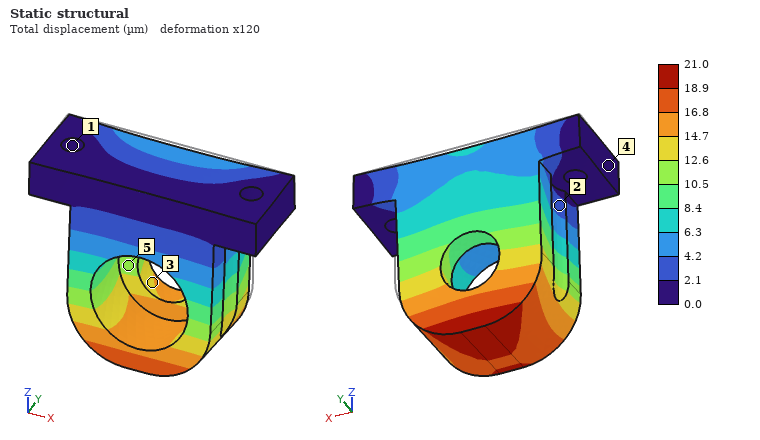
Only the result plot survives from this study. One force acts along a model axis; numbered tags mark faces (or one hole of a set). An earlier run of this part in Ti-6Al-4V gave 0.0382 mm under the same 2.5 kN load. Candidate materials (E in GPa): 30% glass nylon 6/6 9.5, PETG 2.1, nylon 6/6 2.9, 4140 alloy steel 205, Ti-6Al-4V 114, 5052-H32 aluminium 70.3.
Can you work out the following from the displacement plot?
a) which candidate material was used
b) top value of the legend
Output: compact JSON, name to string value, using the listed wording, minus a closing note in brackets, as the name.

{"which candidate material was used": "4140 alloy steel", "top value of the legend": "21.0 µm"}
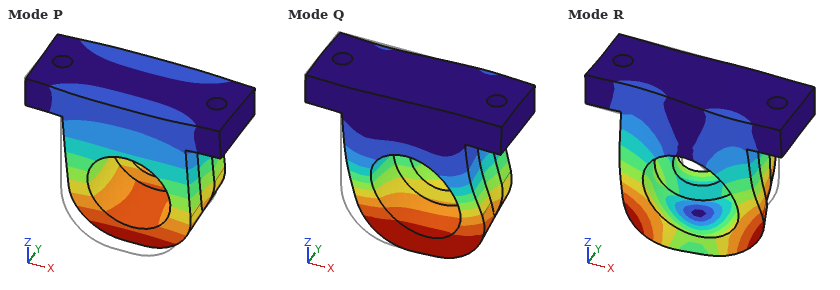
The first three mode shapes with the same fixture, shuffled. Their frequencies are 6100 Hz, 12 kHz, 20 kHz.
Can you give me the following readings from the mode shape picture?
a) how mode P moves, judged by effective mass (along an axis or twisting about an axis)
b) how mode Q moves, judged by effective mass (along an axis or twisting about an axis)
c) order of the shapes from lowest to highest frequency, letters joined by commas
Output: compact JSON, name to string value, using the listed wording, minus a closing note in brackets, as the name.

{"how mode P moves, judged by effective mass": "along Y", "how mode Q moves, judged by effective mass": "along X", "order of the shapes from lowest to highest frequency, letters joined by commas": "P, Q, R"}
